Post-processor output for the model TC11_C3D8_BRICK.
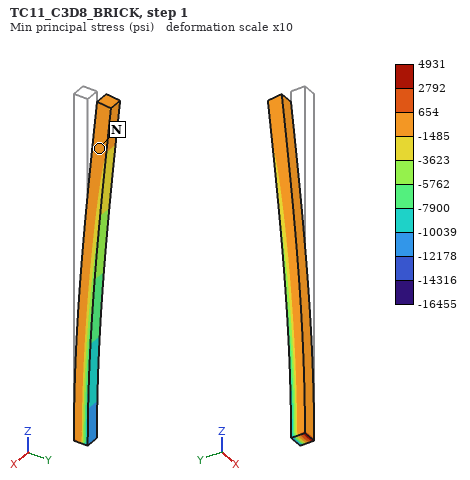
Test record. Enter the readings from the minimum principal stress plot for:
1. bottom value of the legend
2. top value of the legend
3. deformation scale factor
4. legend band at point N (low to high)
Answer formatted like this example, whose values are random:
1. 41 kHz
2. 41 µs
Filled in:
1. -16455 psi
2. 4931 psi
3. 10
4. -1485 to 654 psi
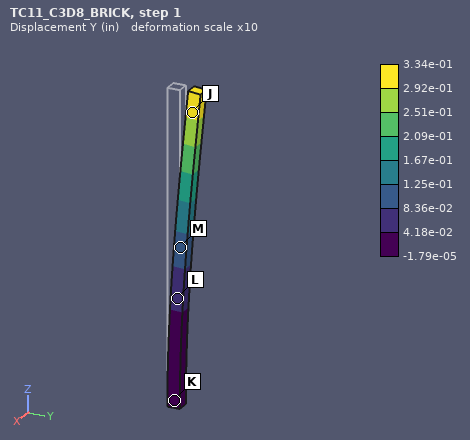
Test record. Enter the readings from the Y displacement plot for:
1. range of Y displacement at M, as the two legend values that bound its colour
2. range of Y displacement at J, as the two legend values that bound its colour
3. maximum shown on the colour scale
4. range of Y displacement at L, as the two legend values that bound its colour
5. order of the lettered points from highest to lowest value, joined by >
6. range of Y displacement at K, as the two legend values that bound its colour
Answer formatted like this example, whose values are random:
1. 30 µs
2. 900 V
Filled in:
1. 8.36e-02 to 1.25e-01 in
2. 2.92e-01 to 3.34e-01 in
3. 3.34e-01 in
4. 4.18e-02 to 8.36e-02 in
5. J > M > L > K
6. -1.79e-05 to 4.18e-02 in
